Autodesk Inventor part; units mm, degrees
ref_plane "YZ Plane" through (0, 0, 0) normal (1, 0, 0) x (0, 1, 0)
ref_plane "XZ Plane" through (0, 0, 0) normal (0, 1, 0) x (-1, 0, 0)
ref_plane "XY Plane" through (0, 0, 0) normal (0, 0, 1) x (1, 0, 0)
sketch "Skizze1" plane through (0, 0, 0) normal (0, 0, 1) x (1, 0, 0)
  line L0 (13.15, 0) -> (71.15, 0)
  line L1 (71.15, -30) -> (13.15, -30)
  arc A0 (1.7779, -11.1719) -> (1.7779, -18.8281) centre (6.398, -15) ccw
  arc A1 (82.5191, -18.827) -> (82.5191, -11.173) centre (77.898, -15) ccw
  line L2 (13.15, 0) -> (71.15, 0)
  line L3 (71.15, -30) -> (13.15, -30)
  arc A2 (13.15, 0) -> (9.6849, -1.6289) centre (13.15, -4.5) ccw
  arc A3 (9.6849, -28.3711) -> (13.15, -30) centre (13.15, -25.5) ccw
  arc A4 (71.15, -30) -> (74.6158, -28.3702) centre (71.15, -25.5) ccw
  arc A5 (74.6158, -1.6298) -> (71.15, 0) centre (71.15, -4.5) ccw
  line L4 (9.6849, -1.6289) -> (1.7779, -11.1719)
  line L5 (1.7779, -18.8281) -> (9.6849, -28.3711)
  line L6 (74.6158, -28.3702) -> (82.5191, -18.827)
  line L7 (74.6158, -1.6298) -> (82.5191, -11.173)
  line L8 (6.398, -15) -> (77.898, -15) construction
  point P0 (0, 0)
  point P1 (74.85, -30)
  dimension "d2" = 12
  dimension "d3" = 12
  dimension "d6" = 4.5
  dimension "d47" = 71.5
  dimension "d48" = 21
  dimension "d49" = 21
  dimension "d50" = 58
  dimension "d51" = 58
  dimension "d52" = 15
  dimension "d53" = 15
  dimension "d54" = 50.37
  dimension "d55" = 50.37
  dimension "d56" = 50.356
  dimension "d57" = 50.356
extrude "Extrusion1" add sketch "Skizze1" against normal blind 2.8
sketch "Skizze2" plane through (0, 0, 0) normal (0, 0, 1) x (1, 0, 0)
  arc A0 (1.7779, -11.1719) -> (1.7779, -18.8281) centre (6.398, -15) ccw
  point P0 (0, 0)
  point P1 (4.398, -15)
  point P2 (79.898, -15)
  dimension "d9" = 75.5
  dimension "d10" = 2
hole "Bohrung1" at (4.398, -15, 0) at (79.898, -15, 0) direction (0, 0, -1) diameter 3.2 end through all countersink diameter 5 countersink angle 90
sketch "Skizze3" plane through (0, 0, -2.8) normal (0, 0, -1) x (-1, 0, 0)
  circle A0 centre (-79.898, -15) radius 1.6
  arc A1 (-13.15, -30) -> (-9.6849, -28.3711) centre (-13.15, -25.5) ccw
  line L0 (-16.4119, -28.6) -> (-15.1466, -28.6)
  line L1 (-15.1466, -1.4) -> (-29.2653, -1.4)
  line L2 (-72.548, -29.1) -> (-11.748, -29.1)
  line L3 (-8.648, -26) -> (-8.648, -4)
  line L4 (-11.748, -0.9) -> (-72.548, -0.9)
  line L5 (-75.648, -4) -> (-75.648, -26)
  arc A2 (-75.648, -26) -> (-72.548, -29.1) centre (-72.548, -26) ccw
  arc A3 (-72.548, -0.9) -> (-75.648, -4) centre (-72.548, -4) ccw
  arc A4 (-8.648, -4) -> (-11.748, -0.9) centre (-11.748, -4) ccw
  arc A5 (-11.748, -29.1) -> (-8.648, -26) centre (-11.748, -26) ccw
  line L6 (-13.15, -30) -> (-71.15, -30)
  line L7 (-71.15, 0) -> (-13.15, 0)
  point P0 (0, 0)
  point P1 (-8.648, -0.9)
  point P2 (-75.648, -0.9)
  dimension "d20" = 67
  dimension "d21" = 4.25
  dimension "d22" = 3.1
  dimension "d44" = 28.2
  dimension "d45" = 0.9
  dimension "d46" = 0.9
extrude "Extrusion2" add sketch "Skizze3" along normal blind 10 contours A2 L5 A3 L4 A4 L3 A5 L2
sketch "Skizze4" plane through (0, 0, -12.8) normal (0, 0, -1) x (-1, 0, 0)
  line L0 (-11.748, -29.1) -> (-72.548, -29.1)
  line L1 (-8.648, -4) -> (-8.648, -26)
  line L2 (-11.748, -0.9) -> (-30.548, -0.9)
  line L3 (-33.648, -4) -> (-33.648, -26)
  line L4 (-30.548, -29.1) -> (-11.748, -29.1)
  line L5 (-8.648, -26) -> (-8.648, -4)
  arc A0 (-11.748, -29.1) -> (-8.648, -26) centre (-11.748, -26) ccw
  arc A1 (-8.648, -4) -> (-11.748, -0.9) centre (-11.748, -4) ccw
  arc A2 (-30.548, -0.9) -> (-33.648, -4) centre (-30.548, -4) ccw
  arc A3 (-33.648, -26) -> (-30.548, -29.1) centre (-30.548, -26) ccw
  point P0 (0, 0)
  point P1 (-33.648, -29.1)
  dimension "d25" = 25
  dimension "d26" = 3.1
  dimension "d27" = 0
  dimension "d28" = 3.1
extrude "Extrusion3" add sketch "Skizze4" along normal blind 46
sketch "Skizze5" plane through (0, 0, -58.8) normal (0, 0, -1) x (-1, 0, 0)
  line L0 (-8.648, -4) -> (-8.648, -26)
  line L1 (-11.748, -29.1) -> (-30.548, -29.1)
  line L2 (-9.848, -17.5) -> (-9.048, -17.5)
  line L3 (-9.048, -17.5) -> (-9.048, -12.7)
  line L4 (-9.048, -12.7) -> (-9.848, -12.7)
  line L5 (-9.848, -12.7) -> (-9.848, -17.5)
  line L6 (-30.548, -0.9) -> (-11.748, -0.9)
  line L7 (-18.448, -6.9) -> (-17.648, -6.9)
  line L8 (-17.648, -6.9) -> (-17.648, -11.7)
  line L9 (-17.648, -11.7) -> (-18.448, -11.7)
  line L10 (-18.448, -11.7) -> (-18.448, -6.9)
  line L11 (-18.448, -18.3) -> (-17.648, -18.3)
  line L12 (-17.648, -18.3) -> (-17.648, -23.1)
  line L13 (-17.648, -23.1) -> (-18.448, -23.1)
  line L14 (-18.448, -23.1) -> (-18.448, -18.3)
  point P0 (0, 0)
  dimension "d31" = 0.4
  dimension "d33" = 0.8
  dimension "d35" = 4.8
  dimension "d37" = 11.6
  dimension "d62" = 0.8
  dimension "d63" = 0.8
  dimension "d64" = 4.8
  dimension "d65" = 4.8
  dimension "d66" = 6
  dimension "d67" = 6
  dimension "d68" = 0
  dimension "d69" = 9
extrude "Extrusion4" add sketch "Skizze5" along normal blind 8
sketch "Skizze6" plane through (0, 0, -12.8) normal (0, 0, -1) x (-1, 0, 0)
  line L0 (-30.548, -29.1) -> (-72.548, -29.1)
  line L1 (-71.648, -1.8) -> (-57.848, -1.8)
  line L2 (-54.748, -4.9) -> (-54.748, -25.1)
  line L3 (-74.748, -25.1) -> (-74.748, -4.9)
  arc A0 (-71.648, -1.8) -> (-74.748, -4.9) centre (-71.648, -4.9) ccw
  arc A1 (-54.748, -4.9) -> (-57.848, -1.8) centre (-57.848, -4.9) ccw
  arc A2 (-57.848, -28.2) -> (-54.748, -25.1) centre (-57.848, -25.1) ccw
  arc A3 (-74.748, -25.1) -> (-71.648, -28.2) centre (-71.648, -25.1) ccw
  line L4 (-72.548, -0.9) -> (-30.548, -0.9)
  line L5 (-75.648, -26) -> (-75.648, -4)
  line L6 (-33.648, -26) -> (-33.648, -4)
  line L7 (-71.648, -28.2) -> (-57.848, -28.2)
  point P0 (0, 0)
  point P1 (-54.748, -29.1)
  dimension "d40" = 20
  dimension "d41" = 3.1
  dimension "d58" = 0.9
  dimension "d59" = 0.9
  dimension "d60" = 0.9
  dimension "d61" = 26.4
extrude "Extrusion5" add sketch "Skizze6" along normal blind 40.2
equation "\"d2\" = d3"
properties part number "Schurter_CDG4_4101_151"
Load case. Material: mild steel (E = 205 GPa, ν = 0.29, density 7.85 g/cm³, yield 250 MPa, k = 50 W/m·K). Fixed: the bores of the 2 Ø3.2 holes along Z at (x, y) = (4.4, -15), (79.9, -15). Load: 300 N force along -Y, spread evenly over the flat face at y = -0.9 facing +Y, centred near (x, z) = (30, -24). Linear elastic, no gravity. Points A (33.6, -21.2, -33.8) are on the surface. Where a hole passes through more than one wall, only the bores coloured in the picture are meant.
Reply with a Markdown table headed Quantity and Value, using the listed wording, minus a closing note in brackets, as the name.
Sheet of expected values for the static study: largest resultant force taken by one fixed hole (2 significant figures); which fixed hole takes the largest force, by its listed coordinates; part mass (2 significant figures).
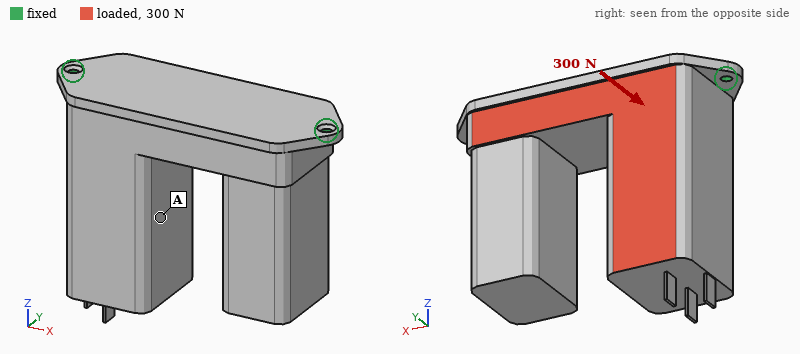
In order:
| Quantity | Value |
|---|---|
| largest resultant force taken by one fixed hole | 200 N |
| which fixed hole takes the largest force, by its listed coordinates | (4.4, -15) |
| part mass | 610 g |
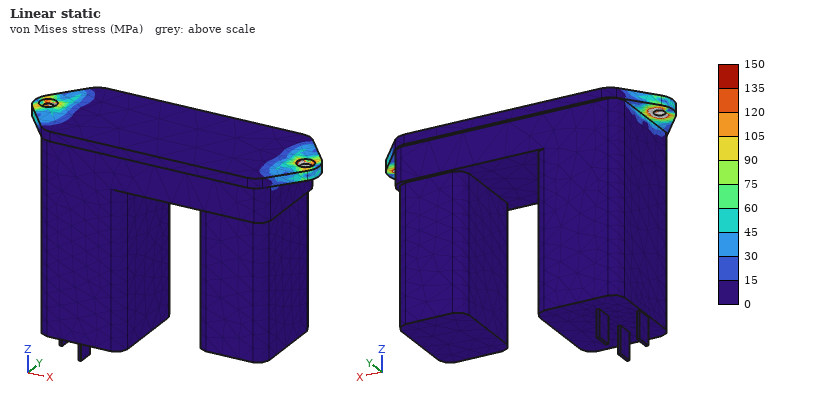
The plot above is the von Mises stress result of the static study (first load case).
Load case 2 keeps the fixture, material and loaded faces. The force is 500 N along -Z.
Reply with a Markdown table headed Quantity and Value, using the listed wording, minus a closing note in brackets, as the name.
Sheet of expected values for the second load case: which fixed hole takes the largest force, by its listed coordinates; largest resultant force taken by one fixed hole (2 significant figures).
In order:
| Quantity | Value |
|---|---|
| which fixed hole takes the largest force, by its listed coordinates | (4.4, -15) |
| largest resultant force taken by one fixed hole | 380 N |
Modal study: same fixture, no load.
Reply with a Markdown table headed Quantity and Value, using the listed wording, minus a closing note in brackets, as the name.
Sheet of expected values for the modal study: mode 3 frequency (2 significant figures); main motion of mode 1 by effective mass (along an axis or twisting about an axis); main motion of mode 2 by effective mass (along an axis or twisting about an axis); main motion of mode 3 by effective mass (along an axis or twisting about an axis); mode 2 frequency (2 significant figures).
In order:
| Quantity | Value |
|---|---|
| mode 3 frequency | 2900 Hz |
| main motion of mode 1 by effective mass | along Y |
| main motion of mode 2 by effective mass | along Z |
| main motion of mode 3 by effective mass | twisting about Z |
| mode 2 frequency | 2300 Hz |
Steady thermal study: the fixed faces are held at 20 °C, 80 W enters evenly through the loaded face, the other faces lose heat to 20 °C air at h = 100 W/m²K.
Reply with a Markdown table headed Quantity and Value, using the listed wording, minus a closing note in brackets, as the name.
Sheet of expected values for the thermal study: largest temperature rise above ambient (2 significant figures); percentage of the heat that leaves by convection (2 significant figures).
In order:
| Quantity | Value |
|---|---|
| largest temperature rise above ambient | 74 K |
| percentage of the heat that leaves by convection | 74 % |
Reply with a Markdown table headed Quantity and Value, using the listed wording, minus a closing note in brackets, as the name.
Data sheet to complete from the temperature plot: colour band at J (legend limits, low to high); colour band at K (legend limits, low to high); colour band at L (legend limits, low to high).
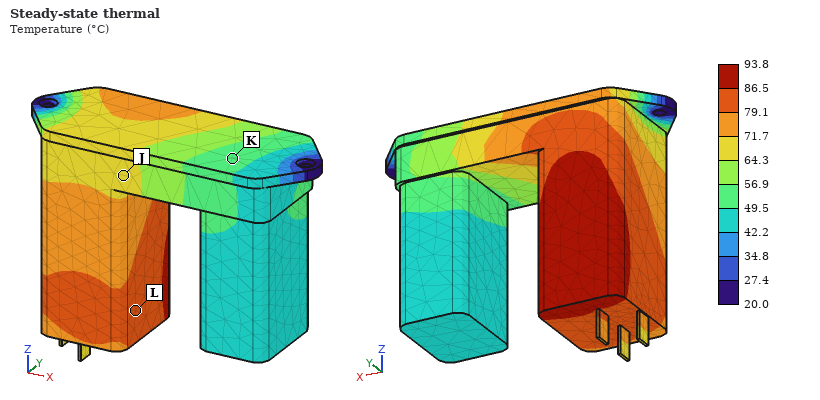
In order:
| Quantity | Value |
|---|---|
| colour band at J | 64.3 to 71.7 °C |
| colour band at K | 49.5 to 56.9 °C |
| colour band at L | 79.1 to 86.5 °C |
